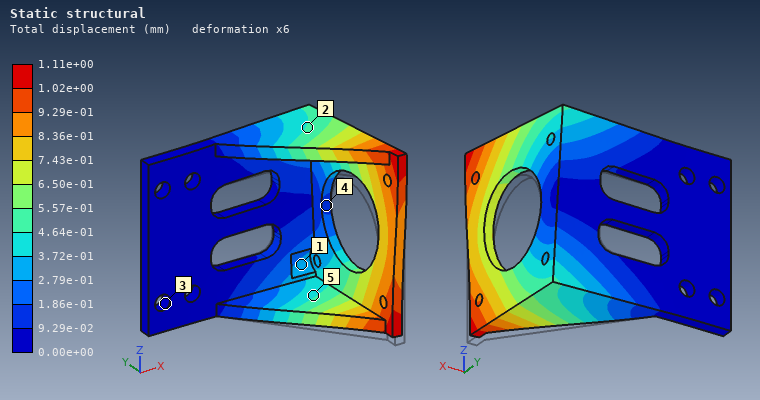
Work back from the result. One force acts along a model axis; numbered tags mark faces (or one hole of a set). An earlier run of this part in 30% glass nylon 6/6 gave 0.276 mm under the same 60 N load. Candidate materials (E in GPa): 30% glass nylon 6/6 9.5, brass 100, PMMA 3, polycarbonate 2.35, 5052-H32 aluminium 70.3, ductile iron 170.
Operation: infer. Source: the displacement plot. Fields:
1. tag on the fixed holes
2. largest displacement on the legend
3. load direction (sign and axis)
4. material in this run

3
1.11e+00 mm
+Z
polycarbonate
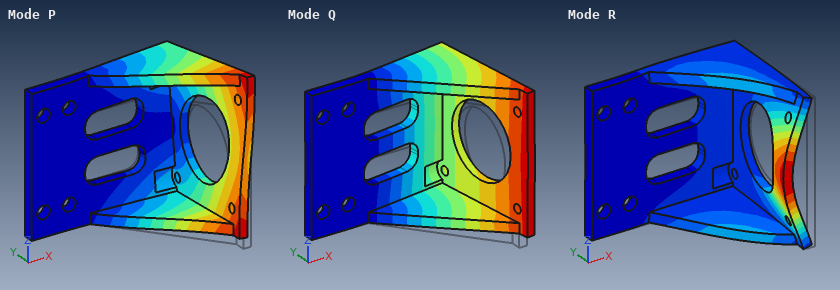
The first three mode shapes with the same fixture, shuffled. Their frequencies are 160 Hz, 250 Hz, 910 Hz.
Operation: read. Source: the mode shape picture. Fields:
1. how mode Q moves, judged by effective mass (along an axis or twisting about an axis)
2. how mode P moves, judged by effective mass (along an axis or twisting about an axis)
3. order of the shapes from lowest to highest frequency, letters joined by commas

along Y
along Z
Q, P, R
